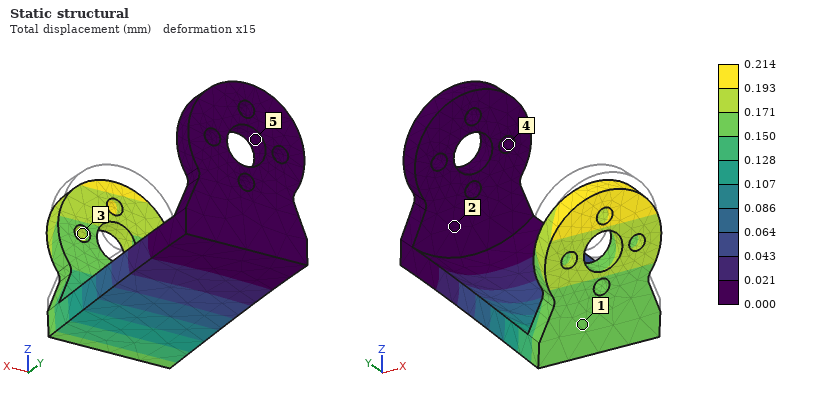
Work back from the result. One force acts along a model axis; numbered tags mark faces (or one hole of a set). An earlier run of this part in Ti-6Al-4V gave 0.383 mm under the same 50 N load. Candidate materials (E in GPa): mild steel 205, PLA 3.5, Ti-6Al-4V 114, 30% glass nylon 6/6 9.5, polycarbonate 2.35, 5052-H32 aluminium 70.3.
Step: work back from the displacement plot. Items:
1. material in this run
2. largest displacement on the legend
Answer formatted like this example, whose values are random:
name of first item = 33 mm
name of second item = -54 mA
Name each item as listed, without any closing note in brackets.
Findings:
material in this run = mild steel
largest displacement on the legend = 0.214 mm
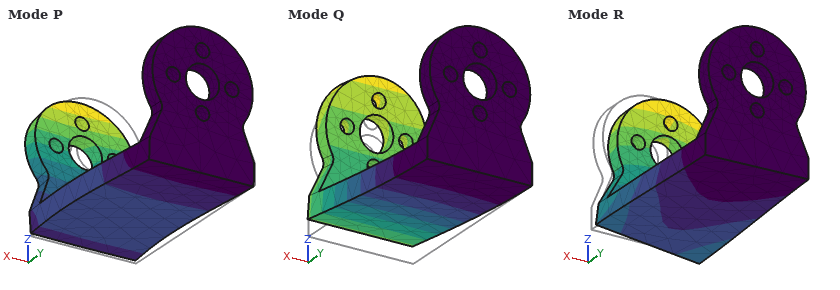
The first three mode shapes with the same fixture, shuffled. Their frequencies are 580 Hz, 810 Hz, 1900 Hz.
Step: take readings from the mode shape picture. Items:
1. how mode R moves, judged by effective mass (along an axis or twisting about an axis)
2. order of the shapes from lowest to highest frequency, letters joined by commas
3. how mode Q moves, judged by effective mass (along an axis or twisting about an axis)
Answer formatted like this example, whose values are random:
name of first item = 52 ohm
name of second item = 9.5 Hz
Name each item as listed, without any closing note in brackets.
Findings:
how mode R moves, judged by effective mass = along X
order of the shapes from lowest to highest frequency, letters joined by commas = Q, R, P
how mode Q moves, judged by effective mass = along Z
